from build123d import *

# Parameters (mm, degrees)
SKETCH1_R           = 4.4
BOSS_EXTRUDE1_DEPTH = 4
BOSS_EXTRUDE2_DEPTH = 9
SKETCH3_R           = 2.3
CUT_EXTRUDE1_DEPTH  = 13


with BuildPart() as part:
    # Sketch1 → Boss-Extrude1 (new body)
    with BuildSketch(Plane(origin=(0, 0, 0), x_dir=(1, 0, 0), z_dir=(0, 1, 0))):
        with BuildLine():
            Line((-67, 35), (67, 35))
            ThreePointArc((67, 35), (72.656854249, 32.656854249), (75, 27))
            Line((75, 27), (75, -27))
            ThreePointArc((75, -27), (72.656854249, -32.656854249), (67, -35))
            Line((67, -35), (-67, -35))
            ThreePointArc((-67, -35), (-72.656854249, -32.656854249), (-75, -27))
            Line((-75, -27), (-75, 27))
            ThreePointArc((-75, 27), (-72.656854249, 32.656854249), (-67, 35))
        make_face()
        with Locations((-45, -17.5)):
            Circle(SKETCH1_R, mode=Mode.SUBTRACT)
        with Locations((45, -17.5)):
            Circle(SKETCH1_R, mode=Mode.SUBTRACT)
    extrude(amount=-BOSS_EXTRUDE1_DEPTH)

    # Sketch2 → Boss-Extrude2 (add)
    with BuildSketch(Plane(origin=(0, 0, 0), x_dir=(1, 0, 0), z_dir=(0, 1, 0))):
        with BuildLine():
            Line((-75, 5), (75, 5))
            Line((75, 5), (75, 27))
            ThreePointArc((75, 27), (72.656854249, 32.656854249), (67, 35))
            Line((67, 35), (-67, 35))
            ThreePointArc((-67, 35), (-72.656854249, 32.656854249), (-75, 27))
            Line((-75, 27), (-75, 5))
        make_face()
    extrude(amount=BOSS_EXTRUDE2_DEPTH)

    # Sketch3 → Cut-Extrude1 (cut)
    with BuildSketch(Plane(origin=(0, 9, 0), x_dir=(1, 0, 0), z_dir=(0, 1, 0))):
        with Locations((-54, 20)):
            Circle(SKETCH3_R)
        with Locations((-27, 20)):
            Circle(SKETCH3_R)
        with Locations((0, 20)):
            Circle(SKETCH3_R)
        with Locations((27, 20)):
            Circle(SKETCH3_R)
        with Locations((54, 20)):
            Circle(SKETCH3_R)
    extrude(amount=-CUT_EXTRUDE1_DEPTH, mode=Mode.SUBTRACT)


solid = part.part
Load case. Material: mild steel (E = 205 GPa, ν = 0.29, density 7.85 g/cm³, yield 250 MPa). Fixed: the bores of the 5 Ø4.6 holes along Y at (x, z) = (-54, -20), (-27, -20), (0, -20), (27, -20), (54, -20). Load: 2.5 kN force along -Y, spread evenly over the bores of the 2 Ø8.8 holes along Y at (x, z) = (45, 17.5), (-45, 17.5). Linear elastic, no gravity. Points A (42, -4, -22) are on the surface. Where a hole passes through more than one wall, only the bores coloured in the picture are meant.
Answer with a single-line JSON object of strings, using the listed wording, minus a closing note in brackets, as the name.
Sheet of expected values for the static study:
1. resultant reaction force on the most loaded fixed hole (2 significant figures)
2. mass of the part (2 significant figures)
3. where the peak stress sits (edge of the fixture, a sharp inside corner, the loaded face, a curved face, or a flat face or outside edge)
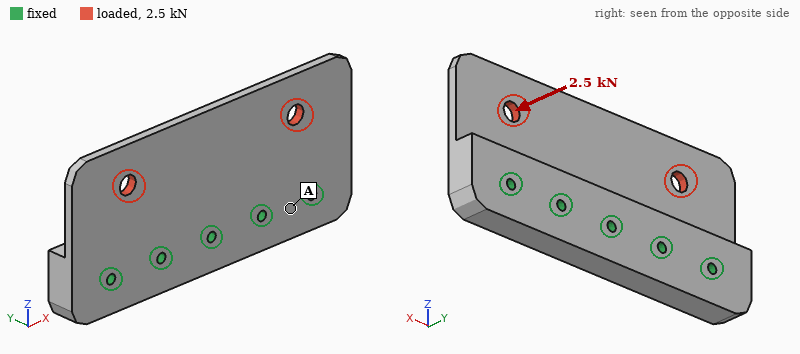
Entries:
{"resultant reaction force on the most loaded fixed hole": "700 N", "mass of the part": "630 g", "where the peak stress sits": "a flat face or outside edge"}
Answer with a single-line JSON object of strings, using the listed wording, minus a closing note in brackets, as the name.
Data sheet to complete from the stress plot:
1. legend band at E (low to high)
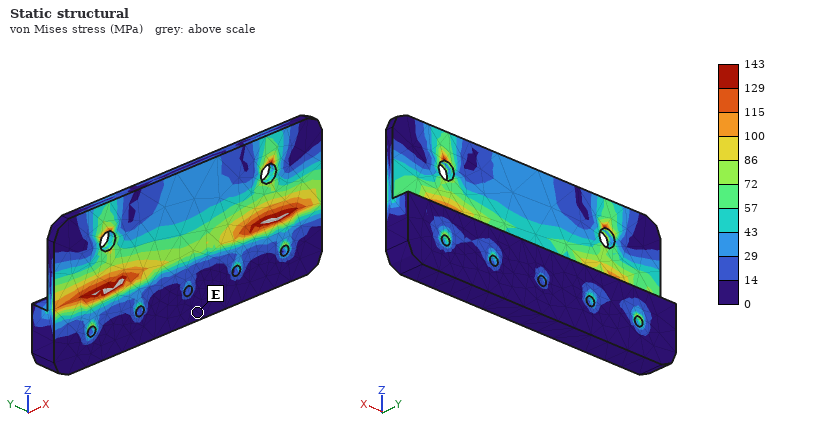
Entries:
{"legend band at E": "0 to 14 MPa"}
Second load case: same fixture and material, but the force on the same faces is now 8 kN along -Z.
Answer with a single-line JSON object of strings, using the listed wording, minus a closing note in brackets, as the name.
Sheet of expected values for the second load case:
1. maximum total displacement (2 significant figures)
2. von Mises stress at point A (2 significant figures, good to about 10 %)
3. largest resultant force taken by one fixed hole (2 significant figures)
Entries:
{"maximum total displacement": "9.1 µm", "von Mises stress at point A": "6.3 MPa", "largest resultant force taken by one fixed hole": "2.5 kN"}
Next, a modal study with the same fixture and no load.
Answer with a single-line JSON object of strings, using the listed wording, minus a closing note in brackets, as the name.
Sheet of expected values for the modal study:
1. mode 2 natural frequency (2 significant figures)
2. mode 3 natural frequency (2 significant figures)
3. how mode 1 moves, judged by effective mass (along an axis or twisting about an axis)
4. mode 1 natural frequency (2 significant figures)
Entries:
{"mode 2 natural frequency": "2200 Hz", "mode 3 natural frequency": "3200 Hz", "how mode 1 moves, judged by effective mass": "along Y", "mode 1 natural frequency": "1900 Hz"}
